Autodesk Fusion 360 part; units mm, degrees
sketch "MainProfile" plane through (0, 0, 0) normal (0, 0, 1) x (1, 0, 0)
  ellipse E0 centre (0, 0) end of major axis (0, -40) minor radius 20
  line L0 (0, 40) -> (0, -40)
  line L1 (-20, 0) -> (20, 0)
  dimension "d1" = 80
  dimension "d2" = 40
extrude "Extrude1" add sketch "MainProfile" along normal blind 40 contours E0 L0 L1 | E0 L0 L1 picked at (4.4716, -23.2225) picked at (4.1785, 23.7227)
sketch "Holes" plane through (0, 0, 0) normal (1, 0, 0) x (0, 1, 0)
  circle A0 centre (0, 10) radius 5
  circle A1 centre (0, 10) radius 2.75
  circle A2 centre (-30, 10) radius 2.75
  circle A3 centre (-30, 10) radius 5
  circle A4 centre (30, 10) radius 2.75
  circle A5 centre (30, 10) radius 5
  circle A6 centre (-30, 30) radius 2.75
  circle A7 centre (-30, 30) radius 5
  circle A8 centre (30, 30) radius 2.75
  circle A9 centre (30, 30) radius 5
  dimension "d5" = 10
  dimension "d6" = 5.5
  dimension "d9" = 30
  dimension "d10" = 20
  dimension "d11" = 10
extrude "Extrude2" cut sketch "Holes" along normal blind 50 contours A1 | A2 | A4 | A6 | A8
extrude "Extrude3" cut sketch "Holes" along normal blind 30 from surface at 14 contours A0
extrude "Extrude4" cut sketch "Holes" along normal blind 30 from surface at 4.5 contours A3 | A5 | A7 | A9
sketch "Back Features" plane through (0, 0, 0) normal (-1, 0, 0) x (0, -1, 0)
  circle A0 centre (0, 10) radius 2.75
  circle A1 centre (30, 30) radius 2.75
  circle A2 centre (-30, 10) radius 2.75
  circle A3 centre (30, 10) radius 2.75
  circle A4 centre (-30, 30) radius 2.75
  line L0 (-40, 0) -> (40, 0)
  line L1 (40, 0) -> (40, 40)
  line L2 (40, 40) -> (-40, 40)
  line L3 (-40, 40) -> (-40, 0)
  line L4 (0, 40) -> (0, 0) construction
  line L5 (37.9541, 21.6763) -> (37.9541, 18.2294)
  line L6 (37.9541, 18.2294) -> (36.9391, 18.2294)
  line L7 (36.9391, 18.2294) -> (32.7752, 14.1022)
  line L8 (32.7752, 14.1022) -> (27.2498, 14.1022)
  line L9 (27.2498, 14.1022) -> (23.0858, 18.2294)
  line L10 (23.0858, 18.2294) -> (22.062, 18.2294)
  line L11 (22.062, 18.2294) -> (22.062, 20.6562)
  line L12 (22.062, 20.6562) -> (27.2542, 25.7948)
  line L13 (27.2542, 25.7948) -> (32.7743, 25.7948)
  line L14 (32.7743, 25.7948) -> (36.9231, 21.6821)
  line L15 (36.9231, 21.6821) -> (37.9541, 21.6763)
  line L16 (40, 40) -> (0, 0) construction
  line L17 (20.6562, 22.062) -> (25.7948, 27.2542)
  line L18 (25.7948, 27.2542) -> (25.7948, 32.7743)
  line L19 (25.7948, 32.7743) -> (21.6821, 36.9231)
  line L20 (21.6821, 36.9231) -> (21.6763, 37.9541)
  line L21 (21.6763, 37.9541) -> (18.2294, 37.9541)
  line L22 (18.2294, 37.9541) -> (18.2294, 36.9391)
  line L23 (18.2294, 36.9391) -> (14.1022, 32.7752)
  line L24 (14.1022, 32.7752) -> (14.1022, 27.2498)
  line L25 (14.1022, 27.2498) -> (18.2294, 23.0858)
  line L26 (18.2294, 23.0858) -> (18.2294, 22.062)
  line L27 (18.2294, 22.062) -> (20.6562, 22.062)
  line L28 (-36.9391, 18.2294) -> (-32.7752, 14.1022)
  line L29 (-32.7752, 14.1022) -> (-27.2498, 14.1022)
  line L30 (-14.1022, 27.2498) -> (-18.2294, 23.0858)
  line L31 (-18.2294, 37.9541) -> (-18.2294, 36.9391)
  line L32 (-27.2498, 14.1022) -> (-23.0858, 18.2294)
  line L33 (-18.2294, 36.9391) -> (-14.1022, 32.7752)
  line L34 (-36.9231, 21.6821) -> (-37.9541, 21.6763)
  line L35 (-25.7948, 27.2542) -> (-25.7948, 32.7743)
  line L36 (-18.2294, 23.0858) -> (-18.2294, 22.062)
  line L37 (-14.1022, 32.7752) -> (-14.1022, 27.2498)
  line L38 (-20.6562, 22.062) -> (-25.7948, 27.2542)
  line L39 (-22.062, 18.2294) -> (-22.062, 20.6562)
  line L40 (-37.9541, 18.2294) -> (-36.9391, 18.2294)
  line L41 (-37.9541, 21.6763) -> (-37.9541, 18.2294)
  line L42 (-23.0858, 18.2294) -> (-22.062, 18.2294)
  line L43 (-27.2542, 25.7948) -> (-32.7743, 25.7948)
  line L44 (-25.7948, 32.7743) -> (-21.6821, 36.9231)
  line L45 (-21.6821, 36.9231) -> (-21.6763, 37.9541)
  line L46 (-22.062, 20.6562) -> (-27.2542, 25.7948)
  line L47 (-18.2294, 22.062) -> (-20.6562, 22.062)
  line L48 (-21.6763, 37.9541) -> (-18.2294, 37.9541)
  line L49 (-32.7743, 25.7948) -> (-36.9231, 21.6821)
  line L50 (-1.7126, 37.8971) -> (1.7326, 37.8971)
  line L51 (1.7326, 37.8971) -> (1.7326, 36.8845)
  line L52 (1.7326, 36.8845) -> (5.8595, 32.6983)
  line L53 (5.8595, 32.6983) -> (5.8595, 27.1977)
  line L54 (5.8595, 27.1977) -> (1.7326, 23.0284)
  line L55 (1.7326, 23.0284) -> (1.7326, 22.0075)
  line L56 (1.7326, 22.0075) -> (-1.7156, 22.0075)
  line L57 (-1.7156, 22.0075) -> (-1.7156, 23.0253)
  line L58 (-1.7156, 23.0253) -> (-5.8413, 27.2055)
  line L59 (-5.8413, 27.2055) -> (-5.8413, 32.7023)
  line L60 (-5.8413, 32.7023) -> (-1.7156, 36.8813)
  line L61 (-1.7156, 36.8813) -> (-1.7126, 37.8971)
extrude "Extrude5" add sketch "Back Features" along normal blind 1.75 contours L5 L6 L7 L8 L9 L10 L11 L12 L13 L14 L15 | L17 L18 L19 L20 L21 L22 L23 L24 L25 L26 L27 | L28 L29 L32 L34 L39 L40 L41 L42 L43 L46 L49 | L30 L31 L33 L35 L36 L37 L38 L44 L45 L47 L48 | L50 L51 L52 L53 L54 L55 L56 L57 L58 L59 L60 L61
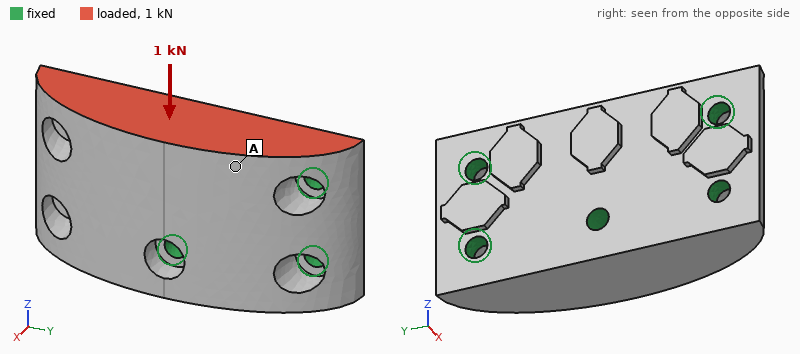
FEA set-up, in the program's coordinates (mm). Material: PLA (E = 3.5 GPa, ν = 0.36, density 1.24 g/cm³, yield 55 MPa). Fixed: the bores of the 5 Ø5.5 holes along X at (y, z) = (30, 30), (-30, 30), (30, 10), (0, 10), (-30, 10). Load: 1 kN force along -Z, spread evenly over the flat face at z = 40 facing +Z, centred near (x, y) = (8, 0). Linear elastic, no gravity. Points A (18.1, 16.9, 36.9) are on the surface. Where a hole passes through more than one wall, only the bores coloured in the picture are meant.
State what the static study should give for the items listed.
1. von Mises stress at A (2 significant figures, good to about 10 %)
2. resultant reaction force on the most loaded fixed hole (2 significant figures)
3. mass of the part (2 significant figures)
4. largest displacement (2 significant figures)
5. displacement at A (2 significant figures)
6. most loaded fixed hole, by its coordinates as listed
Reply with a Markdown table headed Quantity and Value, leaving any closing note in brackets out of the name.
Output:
| Quantity | Value |
|---|---|
| von Mises stress at A | 0.92 MPa |
| resultant reaction force on the most loaded fixed hole | 480 N |
| mass of the part | 59 g |
| largest displacement | 20 µm |
| displacement at A | 17 µm |
| most loaded fixed hole, by its coordinates as listed | (0, 10) |
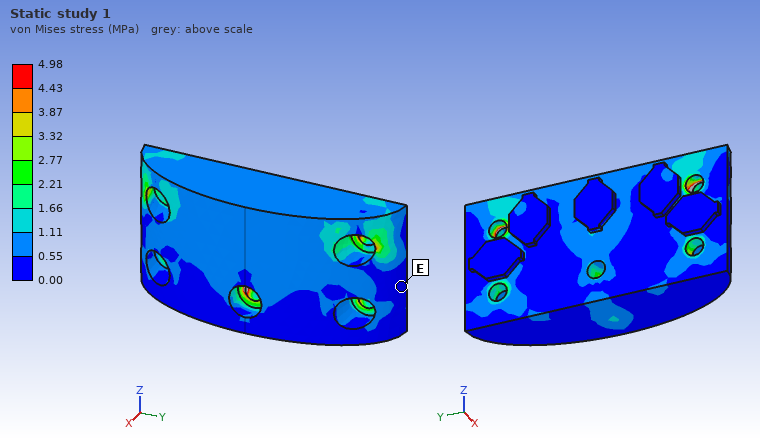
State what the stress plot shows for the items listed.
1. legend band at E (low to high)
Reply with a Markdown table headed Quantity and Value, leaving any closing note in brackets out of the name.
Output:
| Quantity | Value |
|---|---|
| legend band at E | 0.00 to 0.55 MPa |
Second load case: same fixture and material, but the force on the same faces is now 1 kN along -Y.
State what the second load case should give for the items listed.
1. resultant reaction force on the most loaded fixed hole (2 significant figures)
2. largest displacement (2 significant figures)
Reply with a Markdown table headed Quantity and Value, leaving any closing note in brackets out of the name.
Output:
| Quantity | Value |
|---|---|
| resultant reaction force on the most loaded fixed hole | 360 N |
| largest displacement | 25 µm |
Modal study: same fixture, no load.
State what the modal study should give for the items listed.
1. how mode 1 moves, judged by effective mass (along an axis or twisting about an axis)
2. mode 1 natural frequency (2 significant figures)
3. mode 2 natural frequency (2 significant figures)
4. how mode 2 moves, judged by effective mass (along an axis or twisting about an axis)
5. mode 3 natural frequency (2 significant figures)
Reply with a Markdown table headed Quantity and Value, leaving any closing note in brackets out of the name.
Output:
| Quantity | Value |
|---|---|
| how mode 1 moves, judged by effective mass | along X |
| mode 1 natural frequency | 4700 Hz |
| mode 2 natural frequency | 8100 Hz |
| how mode 2 moves, judged by effective mass | along Y |
| mode 3 natural frequency | 8700 Hz |
